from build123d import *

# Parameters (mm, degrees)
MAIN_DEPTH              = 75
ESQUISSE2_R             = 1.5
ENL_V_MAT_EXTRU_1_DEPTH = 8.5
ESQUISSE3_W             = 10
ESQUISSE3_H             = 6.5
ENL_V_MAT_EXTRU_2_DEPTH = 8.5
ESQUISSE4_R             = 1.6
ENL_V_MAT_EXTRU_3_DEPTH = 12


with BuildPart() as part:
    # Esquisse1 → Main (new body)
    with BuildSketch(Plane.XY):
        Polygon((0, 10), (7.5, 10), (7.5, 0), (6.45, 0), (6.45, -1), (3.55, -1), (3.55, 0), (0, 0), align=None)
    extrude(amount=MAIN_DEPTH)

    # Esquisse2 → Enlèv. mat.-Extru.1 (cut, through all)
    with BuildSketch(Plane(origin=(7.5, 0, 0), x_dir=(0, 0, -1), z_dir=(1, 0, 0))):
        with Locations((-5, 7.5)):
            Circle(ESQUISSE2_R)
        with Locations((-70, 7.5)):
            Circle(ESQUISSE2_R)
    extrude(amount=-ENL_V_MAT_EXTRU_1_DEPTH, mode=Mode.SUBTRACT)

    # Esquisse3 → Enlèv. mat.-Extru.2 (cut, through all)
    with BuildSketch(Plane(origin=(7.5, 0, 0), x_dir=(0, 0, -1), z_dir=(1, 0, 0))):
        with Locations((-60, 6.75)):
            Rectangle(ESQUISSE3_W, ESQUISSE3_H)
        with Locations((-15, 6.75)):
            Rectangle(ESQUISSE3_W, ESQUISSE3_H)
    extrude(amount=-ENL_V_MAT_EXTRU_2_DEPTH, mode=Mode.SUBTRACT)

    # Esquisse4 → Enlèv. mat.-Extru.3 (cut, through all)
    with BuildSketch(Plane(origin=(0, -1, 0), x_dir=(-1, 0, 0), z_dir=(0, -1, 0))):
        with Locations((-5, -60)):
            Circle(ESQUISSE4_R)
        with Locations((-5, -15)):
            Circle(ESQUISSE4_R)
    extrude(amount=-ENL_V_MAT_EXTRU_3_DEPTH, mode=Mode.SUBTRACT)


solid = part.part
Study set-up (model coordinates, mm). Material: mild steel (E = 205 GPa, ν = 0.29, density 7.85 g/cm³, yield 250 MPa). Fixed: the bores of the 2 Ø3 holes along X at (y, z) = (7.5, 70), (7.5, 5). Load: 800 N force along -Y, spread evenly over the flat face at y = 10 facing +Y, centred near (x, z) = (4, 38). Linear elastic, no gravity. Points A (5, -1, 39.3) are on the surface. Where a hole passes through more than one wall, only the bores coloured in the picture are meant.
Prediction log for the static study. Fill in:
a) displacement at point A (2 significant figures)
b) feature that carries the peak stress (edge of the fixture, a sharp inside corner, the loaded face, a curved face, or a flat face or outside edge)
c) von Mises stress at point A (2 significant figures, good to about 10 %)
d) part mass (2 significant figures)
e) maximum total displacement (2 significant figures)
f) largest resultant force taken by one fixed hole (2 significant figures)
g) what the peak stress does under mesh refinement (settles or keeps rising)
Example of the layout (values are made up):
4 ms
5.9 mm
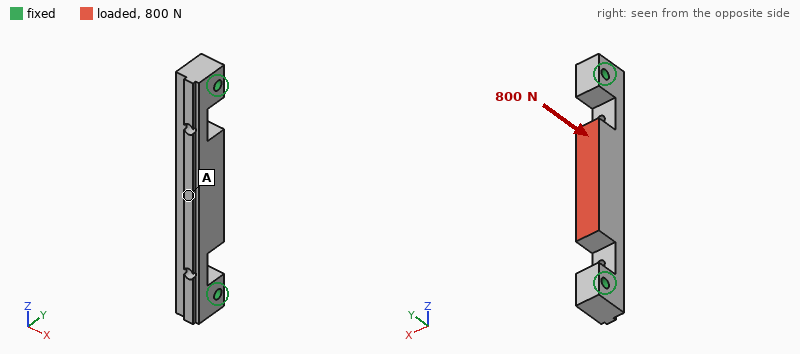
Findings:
26 µm
a sharp inside corner
46 MPa
37 g
26 µm
400 N
keeps rising
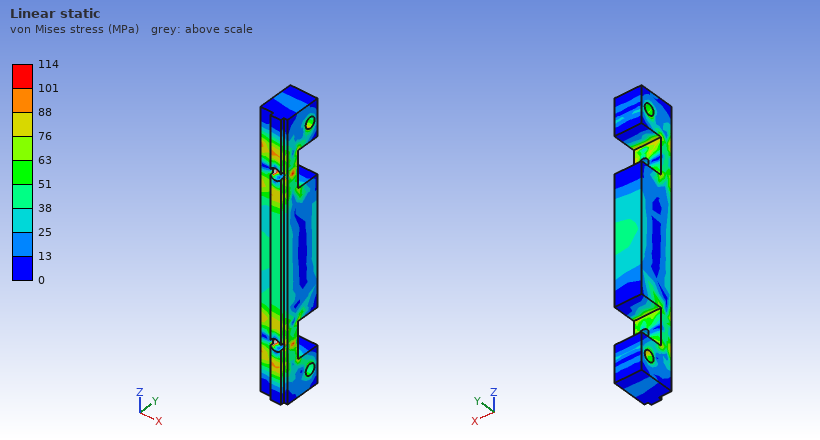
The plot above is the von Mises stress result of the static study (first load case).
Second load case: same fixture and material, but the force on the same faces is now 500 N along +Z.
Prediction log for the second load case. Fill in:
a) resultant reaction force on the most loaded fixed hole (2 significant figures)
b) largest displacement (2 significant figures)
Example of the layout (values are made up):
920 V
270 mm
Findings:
260 N
5.5 µm
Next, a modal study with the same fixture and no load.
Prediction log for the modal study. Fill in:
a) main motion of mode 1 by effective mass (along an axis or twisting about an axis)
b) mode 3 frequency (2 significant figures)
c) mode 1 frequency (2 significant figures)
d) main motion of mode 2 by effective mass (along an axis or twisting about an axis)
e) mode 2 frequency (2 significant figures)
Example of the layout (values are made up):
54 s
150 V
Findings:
along X
11 kHz
5100 Hz
along Y
6100 Hz
